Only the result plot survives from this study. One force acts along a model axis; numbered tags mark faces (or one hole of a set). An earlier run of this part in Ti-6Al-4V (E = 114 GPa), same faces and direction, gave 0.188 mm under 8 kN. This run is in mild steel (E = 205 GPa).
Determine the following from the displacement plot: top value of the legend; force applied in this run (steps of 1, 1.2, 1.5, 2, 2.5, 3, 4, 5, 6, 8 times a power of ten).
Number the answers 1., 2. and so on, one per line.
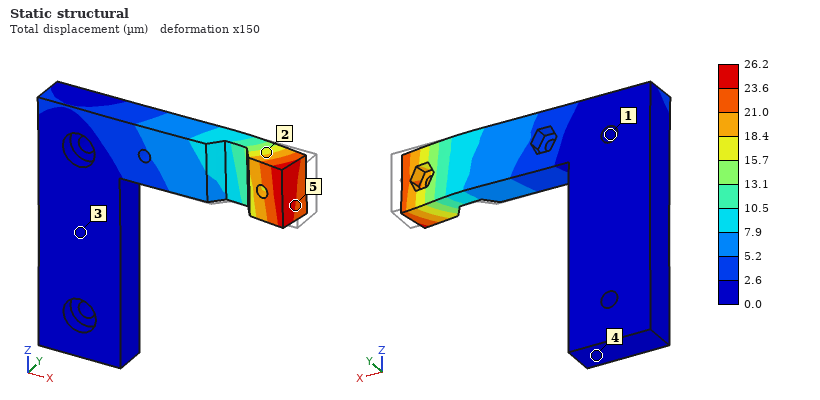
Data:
1. 26.2 µm
2. 2 kN
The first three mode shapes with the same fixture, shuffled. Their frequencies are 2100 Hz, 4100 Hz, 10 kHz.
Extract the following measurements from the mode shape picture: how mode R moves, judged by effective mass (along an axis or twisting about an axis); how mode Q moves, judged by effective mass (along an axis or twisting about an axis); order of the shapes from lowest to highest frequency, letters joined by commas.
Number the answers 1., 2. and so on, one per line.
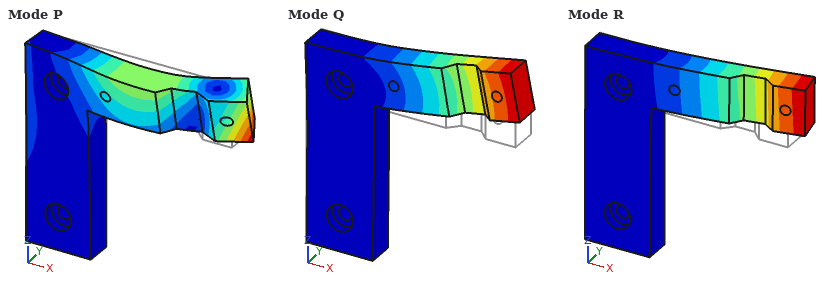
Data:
1. along Y
2. along Z
3. R, Q, P
